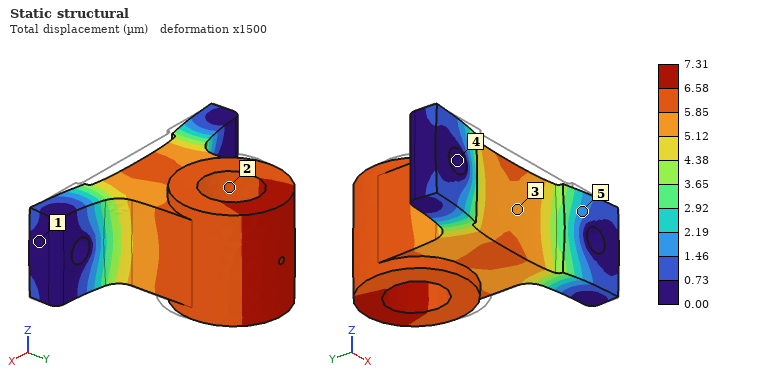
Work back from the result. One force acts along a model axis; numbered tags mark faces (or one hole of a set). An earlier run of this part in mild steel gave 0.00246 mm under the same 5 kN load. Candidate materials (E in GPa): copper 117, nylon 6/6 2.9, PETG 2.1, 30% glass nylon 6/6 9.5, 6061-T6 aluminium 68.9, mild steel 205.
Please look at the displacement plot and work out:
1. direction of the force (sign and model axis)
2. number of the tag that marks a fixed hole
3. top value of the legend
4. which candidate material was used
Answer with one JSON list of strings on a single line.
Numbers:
["+Y", "4", "7.31 µm", "6061-T6 aluminium"]
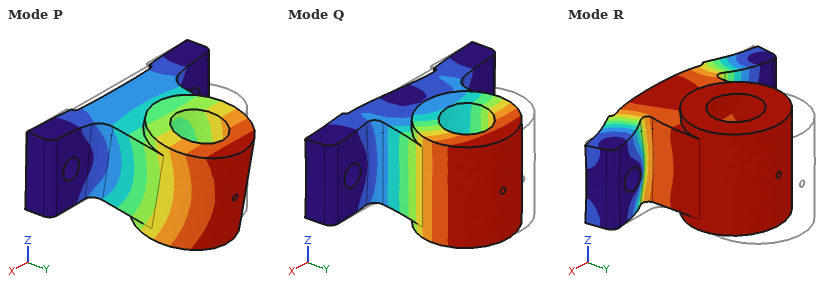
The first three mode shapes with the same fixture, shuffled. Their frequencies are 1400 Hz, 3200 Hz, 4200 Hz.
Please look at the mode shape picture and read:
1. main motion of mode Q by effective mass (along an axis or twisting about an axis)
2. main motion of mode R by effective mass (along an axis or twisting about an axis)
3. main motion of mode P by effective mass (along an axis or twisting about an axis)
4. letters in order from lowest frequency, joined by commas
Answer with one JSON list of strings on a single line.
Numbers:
["along X", "along Y", "along Z", "P, Q, R"]
